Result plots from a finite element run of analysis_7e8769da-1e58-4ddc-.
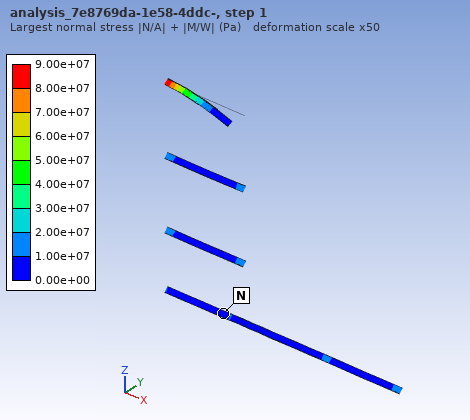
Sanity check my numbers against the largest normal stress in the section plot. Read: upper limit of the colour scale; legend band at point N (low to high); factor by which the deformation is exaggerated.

9.00e+07 Pa
0.00e+00 to 1.00e+07 Pa
50
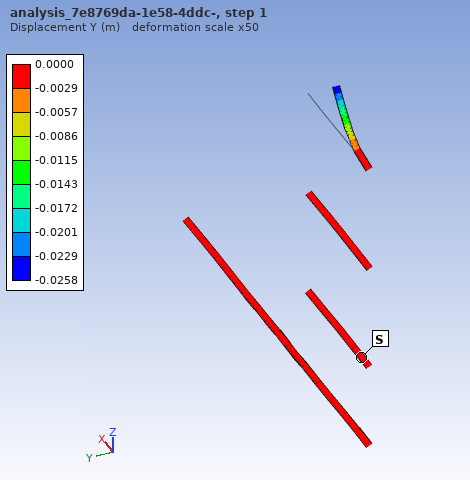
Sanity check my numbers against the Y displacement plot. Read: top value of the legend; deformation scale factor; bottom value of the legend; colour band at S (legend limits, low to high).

0.0000 m
50
-0.0258 m
-0.0029 to 0.0000 m
